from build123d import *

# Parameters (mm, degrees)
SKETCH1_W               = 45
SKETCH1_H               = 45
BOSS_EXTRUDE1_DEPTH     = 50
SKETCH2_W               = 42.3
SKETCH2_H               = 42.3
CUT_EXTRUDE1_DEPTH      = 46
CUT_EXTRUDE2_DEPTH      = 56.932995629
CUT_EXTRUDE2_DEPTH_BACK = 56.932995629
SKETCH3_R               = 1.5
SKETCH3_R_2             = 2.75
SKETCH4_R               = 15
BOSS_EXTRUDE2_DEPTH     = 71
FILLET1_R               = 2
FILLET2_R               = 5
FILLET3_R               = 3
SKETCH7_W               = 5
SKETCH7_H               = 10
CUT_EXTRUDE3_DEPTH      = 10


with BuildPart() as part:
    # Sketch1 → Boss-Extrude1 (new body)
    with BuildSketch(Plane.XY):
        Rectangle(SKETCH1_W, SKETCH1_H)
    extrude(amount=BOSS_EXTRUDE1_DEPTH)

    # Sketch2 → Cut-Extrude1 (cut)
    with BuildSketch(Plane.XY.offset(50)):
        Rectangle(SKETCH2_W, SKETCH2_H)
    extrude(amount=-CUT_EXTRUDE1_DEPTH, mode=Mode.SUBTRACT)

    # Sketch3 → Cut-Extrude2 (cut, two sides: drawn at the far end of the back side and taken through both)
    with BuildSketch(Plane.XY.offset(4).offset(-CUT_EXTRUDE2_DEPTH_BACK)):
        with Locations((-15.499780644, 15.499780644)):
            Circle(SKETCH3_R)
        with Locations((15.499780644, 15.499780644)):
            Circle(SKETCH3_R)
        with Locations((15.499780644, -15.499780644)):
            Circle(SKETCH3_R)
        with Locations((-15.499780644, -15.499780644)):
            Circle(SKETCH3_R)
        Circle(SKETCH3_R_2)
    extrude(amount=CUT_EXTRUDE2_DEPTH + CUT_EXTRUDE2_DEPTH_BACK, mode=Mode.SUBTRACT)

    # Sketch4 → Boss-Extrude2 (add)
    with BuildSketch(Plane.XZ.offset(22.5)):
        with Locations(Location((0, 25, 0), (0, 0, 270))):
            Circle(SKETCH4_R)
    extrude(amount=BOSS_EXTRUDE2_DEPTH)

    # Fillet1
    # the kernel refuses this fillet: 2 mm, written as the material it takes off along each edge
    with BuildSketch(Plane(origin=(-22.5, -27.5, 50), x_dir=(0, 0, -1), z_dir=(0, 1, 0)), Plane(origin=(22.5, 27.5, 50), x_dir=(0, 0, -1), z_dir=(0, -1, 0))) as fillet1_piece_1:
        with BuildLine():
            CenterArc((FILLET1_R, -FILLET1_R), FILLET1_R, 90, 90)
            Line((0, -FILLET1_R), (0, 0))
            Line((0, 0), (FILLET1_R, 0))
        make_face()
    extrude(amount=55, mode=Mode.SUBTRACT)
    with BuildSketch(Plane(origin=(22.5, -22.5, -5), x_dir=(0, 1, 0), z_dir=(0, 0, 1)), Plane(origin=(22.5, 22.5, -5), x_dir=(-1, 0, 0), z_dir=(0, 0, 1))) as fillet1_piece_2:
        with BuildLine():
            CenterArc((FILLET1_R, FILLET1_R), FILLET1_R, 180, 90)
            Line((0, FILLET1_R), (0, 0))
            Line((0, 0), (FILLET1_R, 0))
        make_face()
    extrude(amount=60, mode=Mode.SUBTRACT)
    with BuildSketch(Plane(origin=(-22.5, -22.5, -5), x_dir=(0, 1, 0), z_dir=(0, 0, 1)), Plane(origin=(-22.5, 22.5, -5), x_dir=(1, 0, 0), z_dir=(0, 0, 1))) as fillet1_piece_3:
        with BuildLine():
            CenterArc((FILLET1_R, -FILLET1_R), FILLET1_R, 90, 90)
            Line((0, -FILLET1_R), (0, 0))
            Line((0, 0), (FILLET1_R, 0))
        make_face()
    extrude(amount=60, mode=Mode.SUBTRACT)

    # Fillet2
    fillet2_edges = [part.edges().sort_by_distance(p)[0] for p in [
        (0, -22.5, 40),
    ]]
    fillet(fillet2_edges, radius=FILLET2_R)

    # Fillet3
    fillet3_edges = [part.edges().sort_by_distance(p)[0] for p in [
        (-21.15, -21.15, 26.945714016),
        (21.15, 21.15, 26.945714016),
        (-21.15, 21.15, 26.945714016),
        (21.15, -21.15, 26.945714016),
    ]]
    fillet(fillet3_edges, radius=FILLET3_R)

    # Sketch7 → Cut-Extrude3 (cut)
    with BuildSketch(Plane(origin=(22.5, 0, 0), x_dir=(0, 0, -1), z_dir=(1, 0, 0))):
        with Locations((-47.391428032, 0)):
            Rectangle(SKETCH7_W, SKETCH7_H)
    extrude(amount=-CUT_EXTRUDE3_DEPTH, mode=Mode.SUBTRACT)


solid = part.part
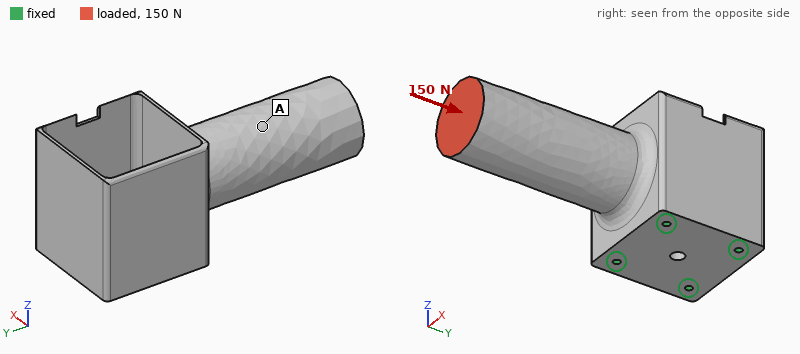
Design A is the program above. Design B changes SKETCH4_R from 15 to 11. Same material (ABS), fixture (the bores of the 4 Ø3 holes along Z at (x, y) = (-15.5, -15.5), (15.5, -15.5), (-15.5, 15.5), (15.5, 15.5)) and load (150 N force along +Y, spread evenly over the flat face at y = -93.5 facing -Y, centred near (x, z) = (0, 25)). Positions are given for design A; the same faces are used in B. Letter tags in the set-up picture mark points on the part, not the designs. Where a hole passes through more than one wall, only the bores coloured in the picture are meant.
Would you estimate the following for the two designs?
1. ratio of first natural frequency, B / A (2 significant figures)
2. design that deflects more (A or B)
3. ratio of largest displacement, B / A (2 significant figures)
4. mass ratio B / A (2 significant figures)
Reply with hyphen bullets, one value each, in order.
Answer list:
- 0.74
- B
- 2.6
- 0.66
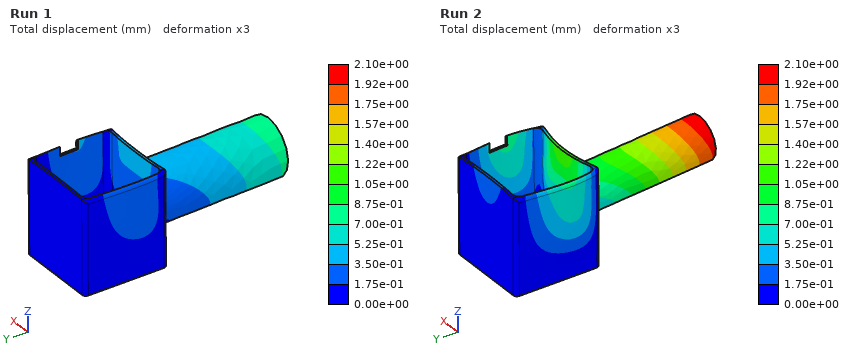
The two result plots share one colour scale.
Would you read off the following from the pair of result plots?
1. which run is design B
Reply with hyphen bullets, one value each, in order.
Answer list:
- Run 2
